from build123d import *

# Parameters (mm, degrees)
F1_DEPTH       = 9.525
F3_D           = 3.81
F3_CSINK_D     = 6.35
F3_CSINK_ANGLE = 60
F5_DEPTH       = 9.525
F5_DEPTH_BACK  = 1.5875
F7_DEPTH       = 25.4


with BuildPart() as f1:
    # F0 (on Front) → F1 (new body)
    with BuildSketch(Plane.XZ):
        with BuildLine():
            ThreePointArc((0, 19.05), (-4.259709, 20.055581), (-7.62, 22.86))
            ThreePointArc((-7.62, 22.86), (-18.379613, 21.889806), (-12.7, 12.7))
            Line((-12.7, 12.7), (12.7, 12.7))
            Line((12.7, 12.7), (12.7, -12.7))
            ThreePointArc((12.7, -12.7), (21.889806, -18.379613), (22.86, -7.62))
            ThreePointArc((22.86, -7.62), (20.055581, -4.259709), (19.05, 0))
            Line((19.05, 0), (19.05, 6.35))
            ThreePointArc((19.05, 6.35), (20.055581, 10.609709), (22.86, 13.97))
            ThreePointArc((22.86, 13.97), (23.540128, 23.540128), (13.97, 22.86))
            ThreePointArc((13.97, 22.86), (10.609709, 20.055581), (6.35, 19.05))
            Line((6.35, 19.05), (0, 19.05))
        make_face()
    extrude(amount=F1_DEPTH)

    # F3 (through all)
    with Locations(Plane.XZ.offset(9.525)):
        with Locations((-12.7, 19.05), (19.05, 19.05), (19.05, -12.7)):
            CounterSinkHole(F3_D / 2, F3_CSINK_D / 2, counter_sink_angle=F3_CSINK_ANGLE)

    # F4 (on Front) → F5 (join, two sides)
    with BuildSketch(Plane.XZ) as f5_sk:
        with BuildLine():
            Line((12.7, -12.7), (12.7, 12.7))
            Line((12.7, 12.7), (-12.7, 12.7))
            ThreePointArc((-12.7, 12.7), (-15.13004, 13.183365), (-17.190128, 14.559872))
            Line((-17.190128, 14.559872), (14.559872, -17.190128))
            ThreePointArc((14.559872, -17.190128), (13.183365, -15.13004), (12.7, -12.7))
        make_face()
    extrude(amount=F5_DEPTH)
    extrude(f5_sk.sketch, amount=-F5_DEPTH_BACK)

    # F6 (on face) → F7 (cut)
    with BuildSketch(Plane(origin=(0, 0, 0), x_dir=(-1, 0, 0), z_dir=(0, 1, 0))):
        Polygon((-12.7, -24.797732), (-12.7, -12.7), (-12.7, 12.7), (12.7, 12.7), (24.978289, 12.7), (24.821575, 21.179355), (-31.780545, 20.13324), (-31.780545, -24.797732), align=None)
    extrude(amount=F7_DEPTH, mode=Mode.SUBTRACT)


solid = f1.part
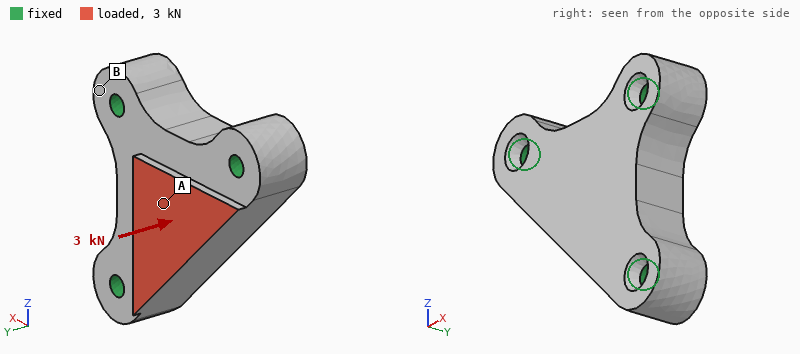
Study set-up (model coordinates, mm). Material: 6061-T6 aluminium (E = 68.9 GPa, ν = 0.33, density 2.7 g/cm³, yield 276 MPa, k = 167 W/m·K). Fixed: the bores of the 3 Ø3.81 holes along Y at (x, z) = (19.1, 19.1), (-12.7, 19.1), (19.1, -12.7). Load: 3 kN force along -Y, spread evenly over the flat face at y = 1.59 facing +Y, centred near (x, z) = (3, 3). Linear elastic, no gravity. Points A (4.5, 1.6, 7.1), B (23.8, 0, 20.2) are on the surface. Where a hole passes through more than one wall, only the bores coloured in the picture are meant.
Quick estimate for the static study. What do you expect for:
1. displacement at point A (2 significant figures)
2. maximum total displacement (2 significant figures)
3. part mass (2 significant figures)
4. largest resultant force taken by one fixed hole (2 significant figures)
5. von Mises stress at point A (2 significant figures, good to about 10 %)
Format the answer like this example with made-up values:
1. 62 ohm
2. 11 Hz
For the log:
1. 14 µm
2. 23 µm
3. 28 g
4. 1.2 kN
5. 21 MPa
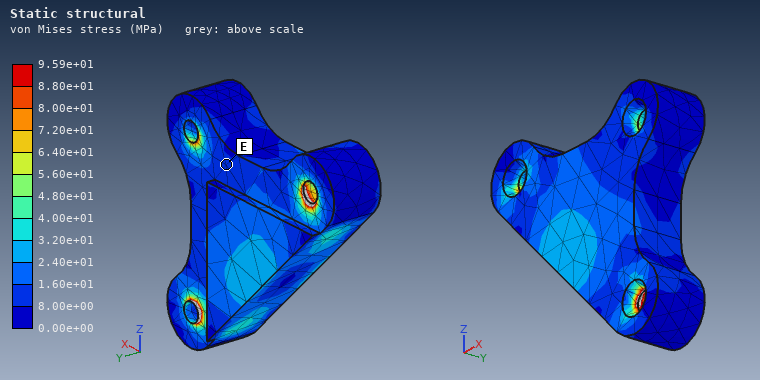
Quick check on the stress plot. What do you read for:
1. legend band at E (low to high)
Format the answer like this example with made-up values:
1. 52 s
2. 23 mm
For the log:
1. 8.00e+00 to 1.60e+01 MPa
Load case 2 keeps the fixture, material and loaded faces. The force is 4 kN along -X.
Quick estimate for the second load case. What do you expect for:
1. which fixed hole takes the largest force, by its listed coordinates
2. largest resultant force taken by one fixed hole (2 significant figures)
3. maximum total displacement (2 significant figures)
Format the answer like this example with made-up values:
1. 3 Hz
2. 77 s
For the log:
1. (19.1, 19.1)
2. 2.0 kN
3. 16 µm
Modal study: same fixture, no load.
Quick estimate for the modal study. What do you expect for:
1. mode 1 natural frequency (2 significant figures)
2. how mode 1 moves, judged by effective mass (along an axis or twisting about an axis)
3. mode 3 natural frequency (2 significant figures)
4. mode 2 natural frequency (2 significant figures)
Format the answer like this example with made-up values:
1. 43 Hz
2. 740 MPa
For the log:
1. 19 kHz
2. along Y
3. 37 kHz
4. 33 kHz
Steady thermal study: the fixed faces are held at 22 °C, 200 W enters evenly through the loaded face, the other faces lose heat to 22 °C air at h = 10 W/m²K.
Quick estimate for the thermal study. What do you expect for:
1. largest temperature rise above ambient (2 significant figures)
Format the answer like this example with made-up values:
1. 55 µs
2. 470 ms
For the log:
1. 60 K
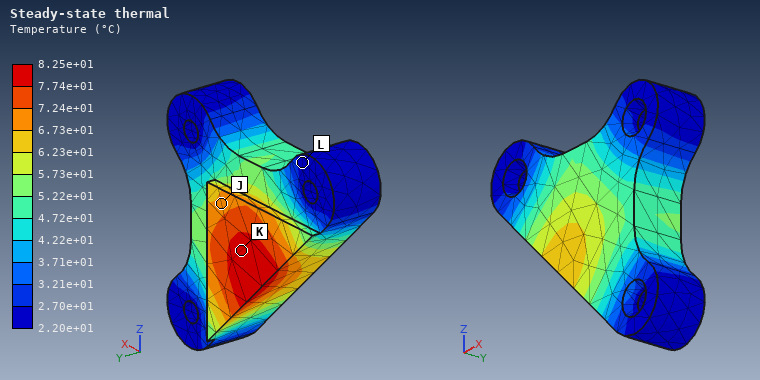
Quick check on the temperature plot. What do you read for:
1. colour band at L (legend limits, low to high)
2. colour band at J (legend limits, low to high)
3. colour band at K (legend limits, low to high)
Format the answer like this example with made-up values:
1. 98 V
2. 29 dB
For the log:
1. 2.20e+01 to 2.70e+01 °C
2. 6.73e+01 to 7.24e+01 °C
3. 7.74e+01 to 8.25e+01 °C
